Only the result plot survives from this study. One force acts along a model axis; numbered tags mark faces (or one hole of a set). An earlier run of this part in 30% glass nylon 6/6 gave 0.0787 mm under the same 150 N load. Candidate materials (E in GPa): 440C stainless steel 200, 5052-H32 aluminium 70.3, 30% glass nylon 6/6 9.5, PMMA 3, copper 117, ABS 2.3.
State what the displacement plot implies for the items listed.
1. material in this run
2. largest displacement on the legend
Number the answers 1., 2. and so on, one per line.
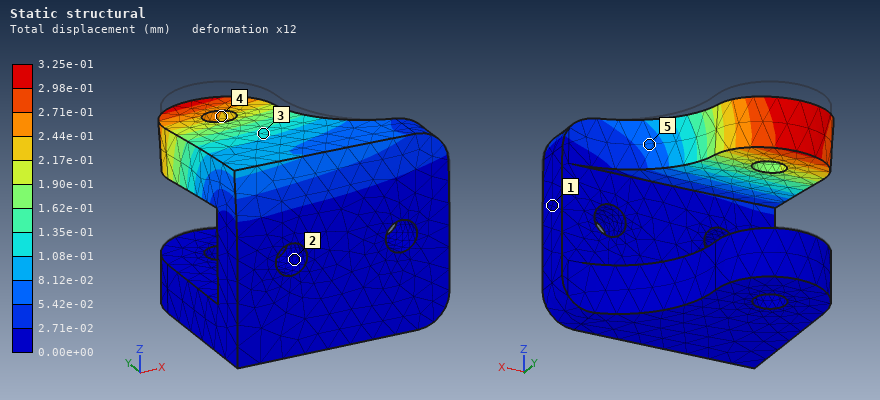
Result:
1. ABS
2. 3.25e-01 mm
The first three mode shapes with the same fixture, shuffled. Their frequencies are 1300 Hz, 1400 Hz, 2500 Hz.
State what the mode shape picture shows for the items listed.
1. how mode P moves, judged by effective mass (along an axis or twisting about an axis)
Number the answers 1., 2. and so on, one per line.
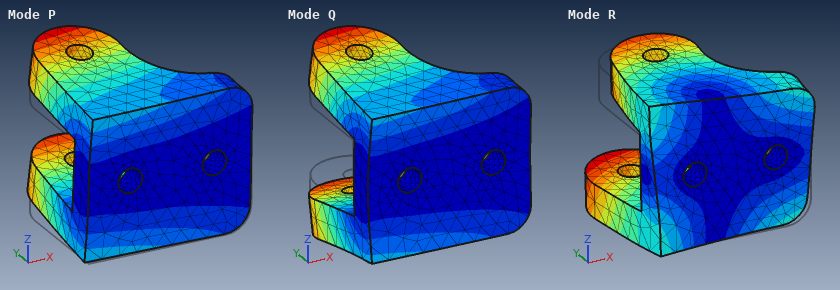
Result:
1. along Z
